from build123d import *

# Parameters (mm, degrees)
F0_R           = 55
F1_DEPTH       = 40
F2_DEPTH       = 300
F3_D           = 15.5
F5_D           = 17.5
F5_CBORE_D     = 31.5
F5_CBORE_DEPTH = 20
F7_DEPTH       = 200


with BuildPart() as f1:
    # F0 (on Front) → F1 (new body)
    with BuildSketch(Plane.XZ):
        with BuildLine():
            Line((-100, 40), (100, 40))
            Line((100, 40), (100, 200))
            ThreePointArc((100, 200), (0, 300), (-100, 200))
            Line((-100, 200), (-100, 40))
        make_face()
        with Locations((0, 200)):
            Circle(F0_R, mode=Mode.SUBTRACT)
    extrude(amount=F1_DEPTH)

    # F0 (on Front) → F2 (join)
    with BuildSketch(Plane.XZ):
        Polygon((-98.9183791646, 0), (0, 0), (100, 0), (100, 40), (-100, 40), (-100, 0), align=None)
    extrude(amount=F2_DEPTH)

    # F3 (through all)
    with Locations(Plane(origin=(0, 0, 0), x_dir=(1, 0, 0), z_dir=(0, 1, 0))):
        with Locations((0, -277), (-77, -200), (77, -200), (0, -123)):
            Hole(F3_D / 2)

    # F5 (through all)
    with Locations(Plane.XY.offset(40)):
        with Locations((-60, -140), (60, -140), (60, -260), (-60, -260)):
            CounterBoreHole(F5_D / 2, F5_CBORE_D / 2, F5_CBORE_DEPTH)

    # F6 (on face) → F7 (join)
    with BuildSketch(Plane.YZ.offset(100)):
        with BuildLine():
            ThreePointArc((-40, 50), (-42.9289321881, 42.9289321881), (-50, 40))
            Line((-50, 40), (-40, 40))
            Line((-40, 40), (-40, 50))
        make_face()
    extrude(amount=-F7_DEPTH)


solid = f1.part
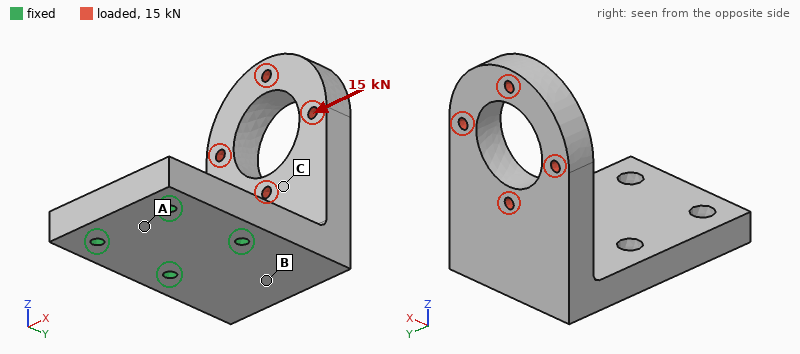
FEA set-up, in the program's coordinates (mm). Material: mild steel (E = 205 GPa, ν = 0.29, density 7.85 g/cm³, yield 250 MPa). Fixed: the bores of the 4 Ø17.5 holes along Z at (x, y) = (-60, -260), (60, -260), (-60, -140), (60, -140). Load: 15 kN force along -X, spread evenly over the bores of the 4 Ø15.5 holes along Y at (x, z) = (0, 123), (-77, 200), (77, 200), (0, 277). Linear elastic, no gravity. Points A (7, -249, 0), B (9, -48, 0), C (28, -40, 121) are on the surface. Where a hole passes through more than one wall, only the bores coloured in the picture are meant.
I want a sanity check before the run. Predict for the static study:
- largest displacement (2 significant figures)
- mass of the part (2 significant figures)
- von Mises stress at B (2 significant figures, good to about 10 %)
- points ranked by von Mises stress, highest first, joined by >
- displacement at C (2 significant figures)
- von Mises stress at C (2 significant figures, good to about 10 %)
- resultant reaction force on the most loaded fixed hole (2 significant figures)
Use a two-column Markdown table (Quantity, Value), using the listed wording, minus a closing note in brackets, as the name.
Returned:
| Quantity | Value |
|---|---|
| largest displacement | 0.21 mm |
| mass of the part | 30 kg |
| von Mises stress at B | 24 MPa |
| points ranked by von Mises stress, highest first, joined by > | B > C > A |
| displacement at C | 0.077 mm |
| von Mises stress at C | 11 MPa |
| resultant reaction force on the most loaded fixed hole | 29 kN |
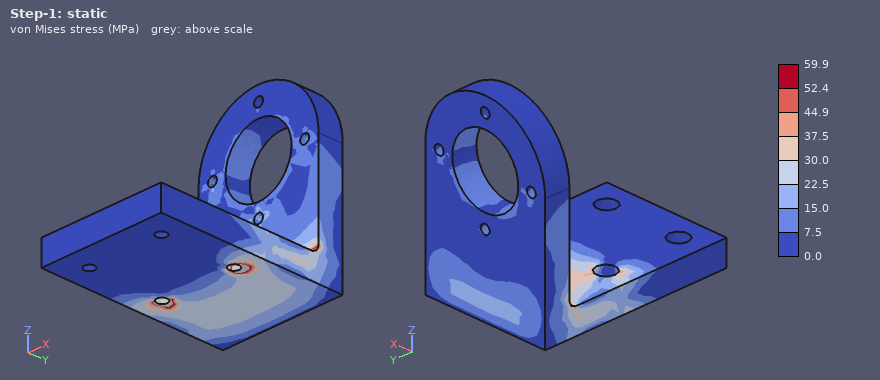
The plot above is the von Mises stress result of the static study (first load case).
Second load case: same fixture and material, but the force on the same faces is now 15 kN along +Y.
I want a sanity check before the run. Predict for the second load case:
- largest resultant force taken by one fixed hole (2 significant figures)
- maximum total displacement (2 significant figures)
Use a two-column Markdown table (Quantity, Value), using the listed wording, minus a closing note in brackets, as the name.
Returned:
| Quantity | Value |
|---|---|
| largest resultant force taken by one fixed hole | 18 kN |
| maximum total displacement | 0.76 mm |
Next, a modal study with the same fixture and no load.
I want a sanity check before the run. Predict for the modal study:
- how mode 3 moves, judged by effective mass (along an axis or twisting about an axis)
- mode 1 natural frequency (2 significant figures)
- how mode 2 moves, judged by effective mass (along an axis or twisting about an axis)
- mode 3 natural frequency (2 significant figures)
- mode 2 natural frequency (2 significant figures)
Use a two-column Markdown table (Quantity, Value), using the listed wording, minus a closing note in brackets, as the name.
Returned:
| Quantity | Value |
|---|---|
| how mode 3 moves, judged by effective mass | along Z |
| mode 1 natural frequency | 300 Hz |
| how mode 2 moves, judged by effective mass | along X |
| mode 3 natural frequency | 910 Hz |
| mode 2 natural frequency | 550 Hz |
